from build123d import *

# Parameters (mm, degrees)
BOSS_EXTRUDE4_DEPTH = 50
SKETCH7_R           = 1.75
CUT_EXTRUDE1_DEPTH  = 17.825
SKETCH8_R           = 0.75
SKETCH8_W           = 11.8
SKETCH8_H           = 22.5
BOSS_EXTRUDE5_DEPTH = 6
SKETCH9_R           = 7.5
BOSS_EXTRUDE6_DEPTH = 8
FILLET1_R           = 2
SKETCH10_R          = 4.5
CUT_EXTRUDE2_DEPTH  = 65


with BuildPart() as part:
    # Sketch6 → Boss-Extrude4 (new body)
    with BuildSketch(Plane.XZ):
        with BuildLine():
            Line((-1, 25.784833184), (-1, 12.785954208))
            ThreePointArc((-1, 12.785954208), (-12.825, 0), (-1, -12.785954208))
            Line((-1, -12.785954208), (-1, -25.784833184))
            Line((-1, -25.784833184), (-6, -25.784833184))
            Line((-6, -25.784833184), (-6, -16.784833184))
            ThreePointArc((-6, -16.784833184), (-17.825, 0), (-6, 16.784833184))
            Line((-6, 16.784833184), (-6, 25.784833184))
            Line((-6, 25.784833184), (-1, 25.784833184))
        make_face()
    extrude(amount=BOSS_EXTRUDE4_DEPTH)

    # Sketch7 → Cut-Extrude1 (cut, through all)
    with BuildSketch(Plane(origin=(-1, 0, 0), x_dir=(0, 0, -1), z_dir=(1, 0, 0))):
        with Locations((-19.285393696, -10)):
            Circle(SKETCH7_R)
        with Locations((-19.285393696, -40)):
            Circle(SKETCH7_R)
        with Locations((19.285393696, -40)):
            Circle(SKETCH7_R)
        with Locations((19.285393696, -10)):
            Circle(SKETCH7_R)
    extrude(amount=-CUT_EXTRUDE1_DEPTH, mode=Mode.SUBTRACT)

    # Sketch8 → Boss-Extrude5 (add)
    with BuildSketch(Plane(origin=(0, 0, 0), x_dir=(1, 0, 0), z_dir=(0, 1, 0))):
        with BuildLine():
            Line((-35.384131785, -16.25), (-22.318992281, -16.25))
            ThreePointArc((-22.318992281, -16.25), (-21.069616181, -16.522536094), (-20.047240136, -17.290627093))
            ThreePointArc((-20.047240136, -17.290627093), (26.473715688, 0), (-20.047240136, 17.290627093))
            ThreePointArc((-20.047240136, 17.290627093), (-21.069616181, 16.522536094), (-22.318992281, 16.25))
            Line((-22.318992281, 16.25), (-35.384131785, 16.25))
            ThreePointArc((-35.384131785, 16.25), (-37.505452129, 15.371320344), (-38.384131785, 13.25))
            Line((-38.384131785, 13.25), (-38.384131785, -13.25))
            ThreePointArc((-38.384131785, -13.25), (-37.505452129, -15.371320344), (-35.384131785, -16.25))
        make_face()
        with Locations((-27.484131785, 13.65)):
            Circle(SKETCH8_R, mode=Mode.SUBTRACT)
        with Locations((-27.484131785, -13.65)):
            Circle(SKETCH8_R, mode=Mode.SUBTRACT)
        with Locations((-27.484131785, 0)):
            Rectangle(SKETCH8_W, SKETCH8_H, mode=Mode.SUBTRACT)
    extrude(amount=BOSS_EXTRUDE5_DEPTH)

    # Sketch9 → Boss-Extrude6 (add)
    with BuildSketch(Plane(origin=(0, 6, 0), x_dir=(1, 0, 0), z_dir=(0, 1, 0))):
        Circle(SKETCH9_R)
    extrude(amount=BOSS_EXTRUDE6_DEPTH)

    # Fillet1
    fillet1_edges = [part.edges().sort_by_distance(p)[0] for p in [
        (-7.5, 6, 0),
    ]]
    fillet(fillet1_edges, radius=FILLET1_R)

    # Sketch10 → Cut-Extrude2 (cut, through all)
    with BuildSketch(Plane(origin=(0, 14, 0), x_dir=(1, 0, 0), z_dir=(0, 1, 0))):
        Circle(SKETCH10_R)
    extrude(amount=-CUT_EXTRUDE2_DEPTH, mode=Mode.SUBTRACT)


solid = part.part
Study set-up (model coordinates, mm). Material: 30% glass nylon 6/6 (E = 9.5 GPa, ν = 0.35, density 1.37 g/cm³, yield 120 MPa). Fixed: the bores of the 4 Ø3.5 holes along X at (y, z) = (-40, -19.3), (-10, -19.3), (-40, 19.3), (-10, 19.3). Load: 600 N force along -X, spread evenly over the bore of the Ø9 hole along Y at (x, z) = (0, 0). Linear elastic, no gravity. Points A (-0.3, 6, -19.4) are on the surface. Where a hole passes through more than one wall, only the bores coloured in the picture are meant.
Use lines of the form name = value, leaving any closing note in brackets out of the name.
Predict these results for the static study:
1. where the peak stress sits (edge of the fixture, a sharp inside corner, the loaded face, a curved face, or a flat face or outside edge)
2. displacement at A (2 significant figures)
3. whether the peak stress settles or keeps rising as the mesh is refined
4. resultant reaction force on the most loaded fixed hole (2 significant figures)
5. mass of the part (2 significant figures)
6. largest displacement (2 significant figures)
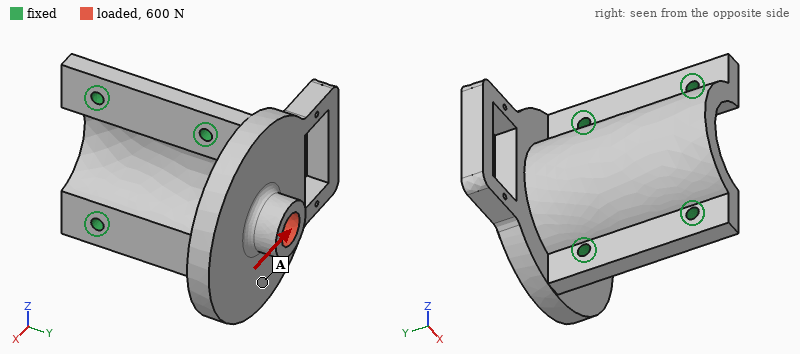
where the peak stress sits = edge of the fixture
displacement at A = 0.074 mm
whether the peak stress settles or keeps rising as the mesh is refined = keeps rising
resultant reaction force on the most loaded fixed hole = 540 N
mass of the part = 42 g
largest displacement = 0.20 mm
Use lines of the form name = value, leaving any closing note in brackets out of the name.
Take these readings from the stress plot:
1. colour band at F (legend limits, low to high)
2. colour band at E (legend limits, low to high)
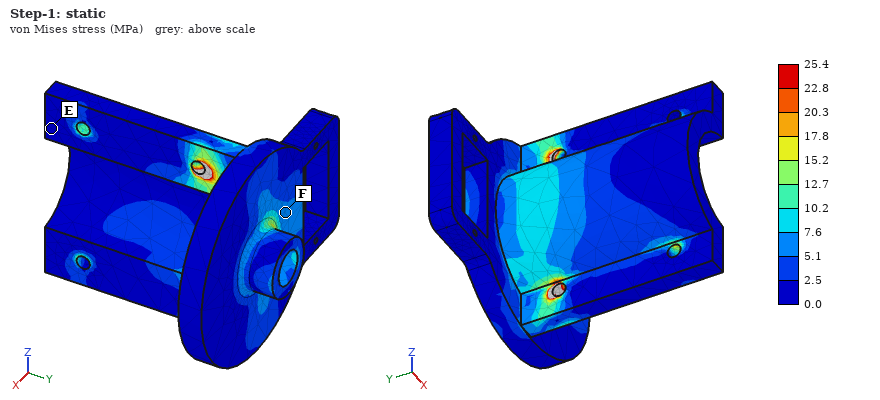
colour band at F = 5.1 to 7.6 MPa
colour band at E = 0.0 to 2.5 MPa
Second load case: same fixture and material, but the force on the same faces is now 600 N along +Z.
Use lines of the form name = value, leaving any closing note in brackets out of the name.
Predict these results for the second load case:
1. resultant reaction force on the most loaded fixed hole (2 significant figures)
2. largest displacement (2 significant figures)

resultant reaction force on the most loaded fixed hole = 370 N
largest displacement = 54 µm
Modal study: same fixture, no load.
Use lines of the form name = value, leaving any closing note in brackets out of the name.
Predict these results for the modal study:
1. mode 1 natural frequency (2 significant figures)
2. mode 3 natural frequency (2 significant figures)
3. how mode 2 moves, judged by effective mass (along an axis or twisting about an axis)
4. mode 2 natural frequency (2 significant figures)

mode 1 natural frequency = 2100 Hz
mode 3 natural frequency = 3500 Hz
how mode 2 moves, judged by effective mass = along Y
mode 2 natural frequency = 3100 Hz
